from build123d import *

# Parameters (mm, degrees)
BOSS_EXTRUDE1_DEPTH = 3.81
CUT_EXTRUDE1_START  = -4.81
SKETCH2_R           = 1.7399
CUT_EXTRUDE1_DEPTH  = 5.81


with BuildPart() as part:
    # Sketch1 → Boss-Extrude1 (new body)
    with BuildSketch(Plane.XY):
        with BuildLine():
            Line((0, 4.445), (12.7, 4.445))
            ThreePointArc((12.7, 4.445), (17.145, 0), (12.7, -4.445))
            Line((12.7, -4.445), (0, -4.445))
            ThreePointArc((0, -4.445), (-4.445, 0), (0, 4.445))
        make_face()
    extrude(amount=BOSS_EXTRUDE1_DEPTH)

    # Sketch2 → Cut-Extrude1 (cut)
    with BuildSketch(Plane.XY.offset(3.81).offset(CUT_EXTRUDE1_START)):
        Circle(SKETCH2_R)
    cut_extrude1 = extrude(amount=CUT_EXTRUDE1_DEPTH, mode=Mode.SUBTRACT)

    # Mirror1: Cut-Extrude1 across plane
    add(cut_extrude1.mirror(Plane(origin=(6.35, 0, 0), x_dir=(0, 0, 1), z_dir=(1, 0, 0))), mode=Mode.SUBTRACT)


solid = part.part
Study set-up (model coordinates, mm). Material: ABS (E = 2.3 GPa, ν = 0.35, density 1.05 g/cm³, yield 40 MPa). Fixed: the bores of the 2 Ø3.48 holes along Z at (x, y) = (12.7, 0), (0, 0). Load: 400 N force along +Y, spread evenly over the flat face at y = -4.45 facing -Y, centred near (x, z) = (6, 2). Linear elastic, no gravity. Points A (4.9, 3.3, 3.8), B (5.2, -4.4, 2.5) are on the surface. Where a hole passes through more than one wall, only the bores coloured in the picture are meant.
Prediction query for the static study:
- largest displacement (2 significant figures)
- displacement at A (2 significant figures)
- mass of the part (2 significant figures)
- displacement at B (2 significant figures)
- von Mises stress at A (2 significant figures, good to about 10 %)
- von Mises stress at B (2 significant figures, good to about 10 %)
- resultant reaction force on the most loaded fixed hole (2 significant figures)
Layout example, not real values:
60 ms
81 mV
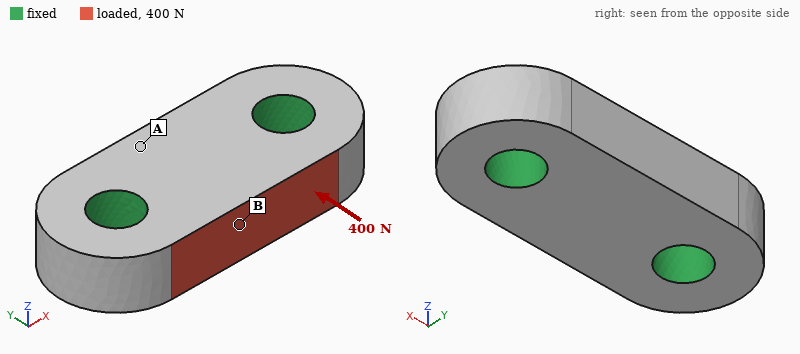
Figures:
33 µm
17 µm
0.62 g
30 µm
3.8 MPa
9.1 MPa
210 N
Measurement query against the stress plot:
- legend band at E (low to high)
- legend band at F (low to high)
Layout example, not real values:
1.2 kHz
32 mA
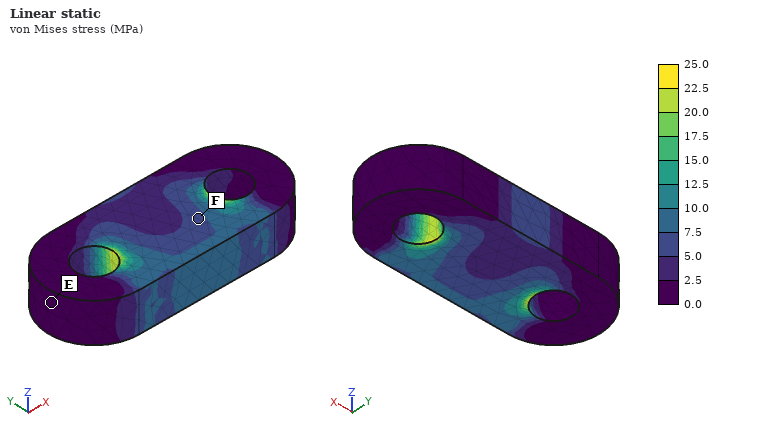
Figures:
0.0 to 2.5 MPa
5.0 to 7.5 MPa
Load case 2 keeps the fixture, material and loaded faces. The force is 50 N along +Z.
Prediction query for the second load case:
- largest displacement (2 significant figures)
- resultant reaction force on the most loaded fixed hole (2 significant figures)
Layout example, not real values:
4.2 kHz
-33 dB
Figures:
22 µm
25 N
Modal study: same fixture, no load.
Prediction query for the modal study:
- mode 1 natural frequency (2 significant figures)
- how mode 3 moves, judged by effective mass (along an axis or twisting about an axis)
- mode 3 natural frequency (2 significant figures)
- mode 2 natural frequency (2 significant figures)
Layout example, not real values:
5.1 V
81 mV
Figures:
29 kHz
along Y
34 kHz
29 kHz
